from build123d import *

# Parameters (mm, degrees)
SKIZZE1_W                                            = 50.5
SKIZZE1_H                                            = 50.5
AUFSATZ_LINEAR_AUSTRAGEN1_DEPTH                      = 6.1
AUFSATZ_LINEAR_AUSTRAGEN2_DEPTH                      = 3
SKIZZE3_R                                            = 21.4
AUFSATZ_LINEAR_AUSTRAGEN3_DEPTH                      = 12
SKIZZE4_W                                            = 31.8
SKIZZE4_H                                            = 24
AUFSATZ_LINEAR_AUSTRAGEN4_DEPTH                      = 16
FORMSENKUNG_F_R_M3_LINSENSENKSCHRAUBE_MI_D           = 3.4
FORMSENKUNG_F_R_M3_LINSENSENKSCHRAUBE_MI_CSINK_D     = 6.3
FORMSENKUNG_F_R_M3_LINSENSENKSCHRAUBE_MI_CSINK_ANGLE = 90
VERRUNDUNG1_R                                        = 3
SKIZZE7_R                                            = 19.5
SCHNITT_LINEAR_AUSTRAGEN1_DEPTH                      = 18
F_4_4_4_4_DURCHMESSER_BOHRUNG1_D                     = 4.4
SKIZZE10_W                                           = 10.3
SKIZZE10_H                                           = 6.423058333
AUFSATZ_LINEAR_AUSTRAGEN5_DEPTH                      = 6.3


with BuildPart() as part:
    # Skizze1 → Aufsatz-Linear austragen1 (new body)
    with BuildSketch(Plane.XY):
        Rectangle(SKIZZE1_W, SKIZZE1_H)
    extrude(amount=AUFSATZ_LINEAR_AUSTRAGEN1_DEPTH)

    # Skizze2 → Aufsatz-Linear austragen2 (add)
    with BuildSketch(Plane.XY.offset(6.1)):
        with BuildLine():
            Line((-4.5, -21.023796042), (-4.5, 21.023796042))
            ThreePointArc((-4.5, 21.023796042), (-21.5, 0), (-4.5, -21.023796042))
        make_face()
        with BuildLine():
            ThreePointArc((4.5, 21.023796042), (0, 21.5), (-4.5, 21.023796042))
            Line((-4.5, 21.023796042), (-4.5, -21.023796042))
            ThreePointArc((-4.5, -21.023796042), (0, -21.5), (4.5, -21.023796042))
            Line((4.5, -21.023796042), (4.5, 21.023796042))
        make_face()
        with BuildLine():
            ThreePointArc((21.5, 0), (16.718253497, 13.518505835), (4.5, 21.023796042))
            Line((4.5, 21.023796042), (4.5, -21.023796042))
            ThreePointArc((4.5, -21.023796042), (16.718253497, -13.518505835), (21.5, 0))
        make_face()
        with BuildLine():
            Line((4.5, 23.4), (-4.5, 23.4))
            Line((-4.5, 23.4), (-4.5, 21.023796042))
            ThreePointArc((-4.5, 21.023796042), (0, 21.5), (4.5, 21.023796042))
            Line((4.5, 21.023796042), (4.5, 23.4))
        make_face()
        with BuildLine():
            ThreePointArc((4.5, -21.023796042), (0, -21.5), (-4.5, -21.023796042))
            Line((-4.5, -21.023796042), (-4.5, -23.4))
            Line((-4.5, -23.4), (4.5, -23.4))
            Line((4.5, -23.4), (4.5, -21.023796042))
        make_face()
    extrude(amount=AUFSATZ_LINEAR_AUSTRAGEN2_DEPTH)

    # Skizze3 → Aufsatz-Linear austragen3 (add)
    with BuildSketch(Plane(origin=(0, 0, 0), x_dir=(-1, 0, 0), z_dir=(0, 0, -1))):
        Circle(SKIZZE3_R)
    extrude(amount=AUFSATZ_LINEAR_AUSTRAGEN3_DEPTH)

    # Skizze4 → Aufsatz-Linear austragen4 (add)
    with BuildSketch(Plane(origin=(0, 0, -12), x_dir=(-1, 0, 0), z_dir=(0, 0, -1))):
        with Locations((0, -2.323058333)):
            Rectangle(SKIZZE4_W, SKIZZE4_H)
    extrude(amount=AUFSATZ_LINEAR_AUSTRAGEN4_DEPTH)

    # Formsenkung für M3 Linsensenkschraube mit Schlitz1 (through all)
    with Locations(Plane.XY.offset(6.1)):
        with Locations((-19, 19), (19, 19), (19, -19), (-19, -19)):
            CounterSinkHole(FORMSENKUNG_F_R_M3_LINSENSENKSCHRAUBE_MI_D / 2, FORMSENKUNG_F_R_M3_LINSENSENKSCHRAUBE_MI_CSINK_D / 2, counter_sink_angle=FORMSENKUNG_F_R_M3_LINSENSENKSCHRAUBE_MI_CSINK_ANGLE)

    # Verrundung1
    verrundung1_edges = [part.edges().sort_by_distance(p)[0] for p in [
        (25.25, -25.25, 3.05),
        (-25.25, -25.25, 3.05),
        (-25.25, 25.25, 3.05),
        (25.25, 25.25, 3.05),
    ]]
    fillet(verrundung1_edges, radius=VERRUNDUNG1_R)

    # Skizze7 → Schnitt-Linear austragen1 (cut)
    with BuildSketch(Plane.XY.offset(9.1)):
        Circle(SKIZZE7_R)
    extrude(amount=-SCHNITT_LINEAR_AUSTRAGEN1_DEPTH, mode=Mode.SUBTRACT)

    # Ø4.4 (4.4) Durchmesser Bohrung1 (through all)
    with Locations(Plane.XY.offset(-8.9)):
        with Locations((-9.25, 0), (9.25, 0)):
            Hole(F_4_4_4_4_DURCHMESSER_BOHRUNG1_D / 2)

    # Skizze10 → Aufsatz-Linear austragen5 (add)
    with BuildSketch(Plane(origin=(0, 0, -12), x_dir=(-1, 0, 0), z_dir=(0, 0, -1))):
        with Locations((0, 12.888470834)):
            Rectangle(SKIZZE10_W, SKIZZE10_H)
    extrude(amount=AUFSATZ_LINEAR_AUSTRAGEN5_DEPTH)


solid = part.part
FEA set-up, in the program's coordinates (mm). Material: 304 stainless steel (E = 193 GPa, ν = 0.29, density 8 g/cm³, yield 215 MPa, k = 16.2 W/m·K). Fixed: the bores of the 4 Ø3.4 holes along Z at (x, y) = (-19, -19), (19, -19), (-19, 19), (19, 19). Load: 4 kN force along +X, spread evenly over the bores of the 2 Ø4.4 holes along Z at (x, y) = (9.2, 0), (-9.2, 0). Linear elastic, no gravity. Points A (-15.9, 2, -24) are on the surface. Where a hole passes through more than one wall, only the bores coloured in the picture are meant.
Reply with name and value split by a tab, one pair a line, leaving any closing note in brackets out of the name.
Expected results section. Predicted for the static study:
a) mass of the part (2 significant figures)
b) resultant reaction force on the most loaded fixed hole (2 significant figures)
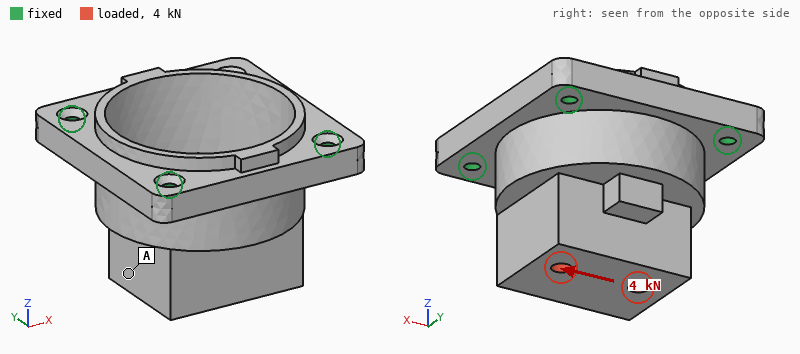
mass of the part	220 g
resultant reaction force on the most loaded fixed hole	1.6 kN
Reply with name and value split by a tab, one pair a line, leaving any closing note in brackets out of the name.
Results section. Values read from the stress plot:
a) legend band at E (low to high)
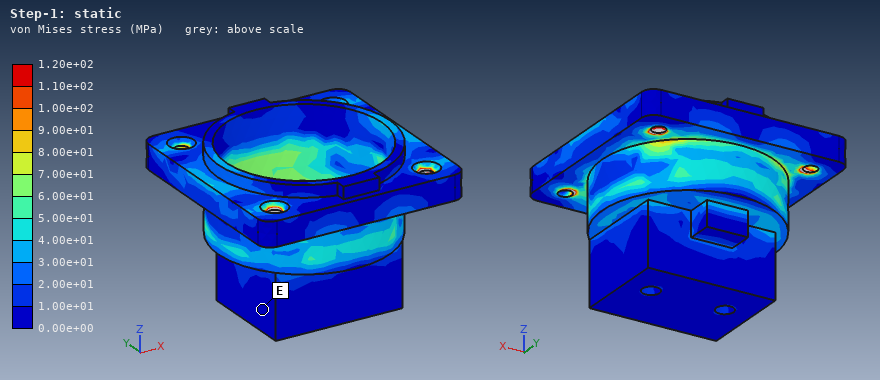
legend band at E	0.00e+00 to 1.00e+01 MPa
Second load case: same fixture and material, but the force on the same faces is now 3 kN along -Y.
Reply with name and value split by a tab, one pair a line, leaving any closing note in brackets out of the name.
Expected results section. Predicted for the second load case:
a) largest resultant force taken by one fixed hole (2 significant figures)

largest resultant force taken by one fixed hole	1.2 kN
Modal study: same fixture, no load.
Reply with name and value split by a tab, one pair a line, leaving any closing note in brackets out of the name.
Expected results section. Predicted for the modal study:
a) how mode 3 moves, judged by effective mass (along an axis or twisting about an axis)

how mode 3 moves, judged by effective mass	along Z
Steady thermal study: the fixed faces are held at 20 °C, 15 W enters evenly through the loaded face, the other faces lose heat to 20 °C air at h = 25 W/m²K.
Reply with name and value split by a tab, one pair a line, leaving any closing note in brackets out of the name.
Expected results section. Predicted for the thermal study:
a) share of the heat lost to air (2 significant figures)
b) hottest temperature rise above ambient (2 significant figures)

share of the heat lost to air	51 %
hottest temperature rise above ambient	57 K
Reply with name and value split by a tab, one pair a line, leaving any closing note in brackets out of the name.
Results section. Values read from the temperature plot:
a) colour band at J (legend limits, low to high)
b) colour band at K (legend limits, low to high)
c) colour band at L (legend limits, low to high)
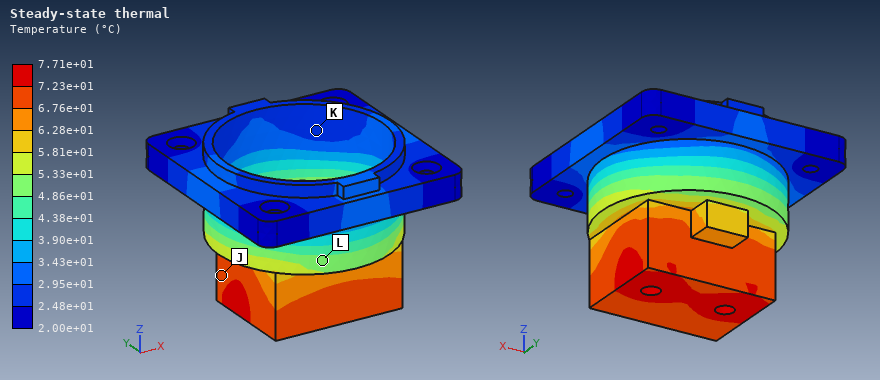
colour band at J	6.76e+01 to 7.23e+01 °C
colour band at K	2.48e+01 to 2.95e+01 °C
colour band at L	4.86e+01 to 5.33e+01 °C
